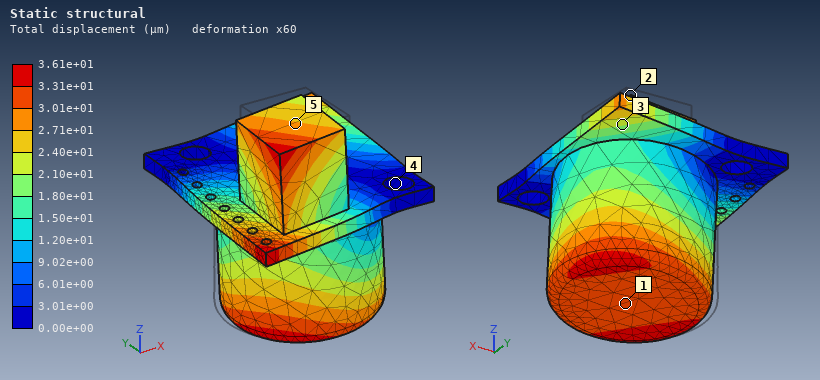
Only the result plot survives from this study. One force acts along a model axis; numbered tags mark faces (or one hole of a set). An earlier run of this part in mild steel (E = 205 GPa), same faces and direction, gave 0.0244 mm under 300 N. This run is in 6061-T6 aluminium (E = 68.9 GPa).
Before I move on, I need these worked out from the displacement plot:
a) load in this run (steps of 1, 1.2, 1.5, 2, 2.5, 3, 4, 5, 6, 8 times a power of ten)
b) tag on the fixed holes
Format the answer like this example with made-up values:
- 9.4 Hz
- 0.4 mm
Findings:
- 150 N
- 4
